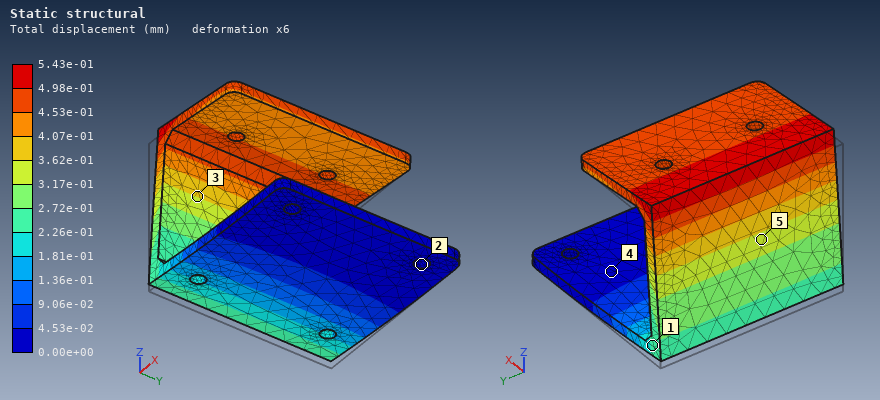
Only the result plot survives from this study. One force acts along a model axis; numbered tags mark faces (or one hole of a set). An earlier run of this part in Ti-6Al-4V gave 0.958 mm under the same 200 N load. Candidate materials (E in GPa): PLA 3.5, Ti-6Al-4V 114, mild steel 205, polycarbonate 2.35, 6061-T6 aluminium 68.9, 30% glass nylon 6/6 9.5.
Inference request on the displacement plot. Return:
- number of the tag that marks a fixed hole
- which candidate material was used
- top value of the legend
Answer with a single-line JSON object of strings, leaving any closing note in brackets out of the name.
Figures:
{"number of the tag that marks a fixed hole": "2", "which candidate material was used": "mild steel", "top value of the legend": "5.43e-01 mm"}
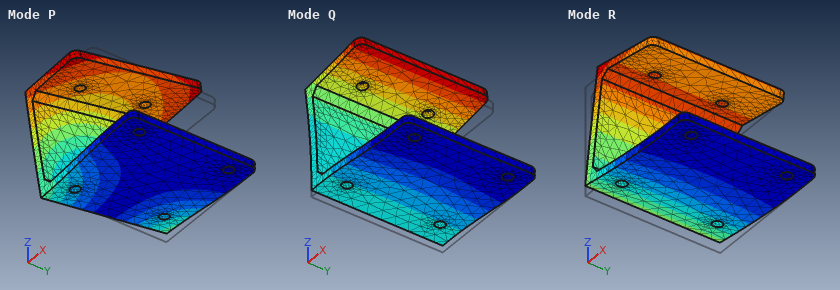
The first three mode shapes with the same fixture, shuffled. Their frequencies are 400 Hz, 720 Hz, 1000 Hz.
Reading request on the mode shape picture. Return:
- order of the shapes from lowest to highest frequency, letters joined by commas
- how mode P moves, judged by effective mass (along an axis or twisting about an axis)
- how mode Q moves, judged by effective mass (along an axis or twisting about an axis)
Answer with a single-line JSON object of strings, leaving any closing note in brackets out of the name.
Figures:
{"order of the shapes from lowest to highest frequency, letters joined by commas": "R, P, Q", "how mode P moves, judged by effective mass": "along Y", "how mode Q moves, judged by effective mass": "along Z"}
